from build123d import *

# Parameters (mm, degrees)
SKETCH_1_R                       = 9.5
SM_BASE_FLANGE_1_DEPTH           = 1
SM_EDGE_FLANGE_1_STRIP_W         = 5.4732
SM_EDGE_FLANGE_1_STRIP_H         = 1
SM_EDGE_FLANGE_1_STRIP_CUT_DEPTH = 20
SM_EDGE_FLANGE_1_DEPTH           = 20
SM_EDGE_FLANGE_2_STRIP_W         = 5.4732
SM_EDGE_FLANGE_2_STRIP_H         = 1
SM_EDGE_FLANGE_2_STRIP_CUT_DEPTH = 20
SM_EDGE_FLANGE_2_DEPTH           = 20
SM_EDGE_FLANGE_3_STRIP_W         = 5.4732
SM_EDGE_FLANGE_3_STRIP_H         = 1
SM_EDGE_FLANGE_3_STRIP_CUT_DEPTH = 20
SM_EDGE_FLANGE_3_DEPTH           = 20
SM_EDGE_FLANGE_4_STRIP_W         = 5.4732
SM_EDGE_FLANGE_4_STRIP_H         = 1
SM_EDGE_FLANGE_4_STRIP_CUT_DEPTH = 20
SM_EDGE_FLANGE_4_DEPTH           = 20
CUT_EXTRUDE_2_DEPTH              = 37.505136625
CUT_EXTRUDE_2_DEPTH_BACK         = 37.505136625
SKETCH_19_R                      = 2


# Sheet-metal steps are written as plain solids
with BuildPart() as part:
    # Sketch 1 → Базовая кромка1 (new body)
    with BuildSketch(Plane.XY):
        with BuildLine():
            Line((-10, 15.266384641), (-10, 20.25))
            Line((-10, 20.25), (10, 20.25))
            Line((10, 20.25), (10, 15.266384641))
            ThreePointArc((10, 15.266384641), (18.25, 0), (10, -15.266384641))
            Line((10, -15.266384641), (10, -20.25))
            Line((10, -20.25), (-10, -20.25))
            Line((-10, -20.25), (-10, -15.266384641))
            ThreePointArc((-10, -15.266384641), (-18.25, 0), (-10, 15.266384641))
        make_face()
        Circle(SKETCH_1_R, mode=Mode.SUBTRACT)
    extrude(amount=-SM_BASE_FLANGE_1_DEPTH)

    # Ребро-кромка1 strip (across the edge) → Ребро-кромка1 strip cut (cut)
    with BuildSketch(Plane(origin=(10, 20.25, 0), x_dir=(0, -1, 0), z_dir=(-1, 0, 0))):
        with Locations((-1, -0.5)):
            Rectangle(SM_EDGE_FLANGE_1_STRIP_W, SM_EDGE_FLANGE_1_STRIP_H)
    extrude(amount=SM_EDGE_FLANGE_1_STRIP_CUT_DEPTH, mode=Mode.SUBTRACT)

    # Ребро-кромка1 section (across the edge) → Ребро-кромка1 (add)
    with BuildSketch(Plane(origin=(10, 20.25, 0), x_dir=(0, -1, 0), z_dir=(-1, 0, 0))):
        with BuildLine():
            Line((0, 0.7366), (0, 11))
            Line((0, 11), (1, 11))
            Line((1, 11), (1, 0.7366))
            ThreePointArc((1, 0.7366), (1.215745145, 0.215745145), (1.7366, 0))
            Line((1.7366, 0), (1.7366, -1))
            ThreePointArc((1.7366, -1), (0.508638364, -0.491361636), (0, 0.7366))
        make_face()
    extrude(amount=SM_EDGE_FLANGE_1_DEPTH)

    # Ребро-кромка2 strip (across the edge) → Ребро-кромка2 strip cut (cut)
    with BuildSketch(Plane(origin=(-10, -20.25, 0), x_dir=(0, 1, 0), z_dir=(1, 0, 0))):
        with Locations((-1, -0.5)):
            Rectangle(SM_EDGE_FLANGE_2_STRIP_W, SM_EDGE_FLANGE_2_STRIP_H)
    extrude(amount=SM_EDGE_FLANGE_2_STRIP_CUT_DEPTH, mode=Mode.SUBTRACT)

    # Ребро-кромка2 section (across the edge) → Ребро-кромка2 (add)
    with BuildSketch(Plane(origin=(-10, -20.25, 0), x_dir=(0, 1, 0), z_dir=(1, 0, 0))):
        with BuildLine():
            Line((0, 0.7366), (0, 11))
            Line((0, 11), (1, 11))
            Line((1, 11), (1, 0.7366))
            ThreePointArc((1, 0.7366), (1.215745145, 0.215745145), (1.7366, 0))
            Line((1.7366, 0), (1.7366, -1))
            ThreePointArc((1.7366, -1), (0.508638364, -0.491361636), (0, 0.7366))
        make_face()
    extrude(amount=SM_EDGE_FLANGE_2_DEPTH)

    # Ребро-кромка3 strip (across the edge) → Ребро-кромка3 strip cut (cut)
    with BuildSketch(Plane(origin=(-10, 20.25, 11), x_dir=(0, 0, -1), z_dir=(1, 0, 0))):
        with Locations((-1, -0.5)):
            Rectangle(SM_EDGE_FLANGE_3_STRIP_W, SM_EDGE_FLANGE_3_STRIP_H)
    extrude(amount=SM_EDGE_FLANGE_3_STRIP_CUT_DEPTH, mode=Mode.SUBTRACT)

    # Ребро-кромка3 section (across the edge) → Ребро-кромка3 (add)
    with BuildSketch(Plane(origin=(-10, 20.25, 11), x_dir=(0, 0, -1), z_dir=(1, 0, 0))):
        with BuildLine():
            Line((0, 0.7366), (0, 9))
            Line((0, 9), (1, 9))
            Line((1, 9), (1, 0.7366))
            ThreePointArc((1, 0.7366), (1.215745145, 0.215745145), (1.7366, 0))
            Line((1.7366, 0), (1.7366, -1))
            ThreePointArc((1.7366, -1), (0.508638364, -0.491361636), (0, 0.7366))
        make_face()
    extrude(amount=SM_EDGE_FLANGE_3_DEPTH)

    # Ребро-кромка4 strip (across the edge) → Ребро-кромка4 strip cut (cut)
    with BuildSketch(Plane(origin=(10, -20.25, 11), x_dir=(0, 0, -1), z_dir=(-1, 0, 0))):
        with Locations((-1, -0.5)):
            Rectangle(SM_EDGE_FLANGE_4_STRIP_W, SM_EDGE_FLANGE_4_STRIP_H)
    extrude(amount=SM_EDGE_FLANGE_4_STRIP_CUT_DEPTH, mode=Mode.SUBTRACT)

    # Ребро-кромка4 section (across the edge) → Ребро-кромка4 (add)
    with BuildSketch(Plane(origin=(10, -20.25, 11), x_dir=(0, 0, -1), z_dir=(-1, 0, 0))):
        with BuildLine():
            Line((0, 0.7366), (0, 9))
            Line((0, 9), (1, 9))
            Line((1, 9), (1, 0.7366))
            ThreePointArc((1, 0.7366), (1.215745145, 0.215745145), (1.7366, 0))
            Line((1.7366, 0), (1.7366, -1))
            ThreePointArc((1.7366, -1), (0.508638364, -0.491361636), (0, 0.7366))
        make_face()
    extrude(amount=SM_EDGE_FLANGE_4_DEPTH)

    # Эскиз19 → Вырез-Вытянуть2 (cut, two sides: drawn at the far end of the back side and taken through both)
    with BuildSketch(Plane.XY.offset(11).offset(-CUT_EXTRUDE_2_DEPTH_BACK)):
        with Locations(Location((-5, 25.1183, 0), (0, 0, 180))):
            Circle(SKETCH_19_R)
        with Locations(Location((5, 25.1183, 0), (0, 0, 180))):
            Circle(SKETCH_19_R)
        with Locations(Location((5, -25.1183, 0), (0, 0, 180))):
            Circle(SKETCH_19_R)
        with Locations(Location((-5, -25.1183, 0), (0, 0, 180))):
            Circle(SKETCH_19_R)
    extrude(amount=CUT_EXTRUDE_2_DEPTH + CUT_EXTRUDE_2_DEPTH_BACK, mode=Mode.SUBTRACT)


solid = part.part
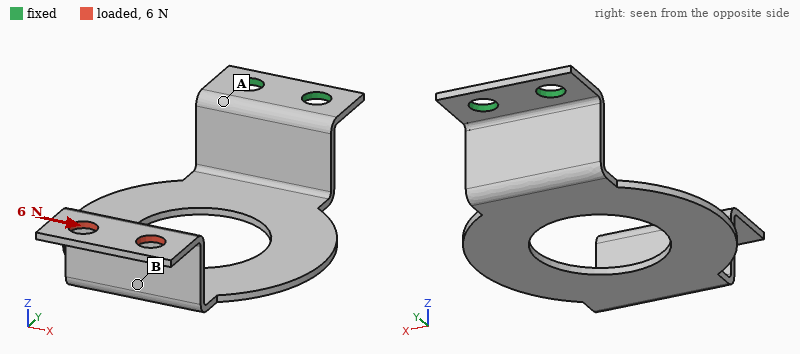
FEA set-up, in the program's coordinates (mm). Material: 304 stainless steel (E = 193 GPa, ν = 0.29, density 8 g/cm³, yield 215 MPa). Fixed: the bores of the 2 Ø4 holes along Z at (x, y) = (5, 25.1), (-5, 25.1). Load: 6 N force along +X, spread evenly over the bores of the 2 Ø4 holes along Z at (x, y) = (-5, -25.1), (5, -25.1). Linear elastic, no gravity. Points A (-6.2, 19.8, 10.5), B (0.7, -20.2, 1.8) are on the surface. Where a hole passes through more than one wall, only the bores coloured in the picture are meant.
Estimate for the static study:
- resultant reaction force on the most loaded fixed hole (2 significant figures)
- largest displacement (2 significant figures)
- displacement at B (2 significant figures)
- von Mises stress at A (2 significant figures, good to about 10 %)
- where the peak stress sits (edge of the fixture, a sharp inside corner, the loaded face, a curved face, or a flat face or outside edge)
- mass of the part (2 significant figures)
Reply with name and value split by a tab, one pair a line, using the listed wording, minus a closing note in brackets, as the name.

resultant reaction force on the most loaded fixed hole	22 N
largest displacement	0.27 mm
displacement at B	0.16 mm
von Mises stress at A	34 MPa
where the peak stress sits	a curved face
mass of the part	13 g
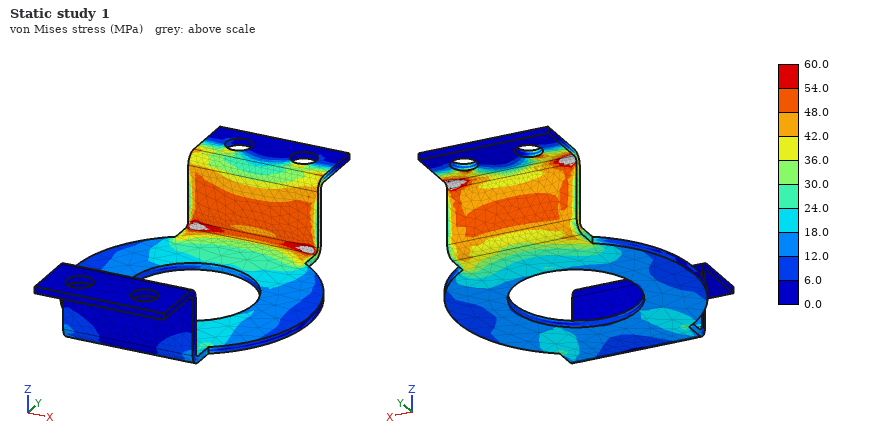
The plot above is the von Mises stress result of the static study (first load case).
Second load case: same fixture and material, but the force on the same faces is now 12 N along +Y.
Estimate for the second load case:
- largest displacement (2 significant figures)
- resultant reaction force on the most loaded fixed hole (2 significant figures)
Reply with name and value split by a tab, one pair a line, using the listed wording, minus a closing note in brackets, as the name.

largest displacement	0.67 mm
resultant reaction force on the most loaded fixed hole	6.1 N
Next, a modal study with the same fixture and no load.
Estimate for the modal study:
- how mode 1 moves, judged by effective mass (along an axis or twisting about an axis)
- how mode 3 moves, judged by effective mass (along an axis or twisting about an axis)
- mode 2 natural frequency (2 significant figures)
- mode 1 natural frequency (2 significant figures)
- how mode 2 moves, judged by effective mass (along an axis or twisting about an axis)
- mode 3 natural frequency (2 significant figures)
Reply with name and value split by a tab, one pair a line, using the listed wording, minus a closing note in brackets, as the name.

how mode 1 moves, judged by effective mass	along Z
how mode 3 moves, judged by effective mass	along Y
mode 2 natural frequency	420 Hz
mode 1 natural frequency	190 Hz
how mode 2 moves, judged by effective mass	along X
mode 3 natural frequency	860 Hz
